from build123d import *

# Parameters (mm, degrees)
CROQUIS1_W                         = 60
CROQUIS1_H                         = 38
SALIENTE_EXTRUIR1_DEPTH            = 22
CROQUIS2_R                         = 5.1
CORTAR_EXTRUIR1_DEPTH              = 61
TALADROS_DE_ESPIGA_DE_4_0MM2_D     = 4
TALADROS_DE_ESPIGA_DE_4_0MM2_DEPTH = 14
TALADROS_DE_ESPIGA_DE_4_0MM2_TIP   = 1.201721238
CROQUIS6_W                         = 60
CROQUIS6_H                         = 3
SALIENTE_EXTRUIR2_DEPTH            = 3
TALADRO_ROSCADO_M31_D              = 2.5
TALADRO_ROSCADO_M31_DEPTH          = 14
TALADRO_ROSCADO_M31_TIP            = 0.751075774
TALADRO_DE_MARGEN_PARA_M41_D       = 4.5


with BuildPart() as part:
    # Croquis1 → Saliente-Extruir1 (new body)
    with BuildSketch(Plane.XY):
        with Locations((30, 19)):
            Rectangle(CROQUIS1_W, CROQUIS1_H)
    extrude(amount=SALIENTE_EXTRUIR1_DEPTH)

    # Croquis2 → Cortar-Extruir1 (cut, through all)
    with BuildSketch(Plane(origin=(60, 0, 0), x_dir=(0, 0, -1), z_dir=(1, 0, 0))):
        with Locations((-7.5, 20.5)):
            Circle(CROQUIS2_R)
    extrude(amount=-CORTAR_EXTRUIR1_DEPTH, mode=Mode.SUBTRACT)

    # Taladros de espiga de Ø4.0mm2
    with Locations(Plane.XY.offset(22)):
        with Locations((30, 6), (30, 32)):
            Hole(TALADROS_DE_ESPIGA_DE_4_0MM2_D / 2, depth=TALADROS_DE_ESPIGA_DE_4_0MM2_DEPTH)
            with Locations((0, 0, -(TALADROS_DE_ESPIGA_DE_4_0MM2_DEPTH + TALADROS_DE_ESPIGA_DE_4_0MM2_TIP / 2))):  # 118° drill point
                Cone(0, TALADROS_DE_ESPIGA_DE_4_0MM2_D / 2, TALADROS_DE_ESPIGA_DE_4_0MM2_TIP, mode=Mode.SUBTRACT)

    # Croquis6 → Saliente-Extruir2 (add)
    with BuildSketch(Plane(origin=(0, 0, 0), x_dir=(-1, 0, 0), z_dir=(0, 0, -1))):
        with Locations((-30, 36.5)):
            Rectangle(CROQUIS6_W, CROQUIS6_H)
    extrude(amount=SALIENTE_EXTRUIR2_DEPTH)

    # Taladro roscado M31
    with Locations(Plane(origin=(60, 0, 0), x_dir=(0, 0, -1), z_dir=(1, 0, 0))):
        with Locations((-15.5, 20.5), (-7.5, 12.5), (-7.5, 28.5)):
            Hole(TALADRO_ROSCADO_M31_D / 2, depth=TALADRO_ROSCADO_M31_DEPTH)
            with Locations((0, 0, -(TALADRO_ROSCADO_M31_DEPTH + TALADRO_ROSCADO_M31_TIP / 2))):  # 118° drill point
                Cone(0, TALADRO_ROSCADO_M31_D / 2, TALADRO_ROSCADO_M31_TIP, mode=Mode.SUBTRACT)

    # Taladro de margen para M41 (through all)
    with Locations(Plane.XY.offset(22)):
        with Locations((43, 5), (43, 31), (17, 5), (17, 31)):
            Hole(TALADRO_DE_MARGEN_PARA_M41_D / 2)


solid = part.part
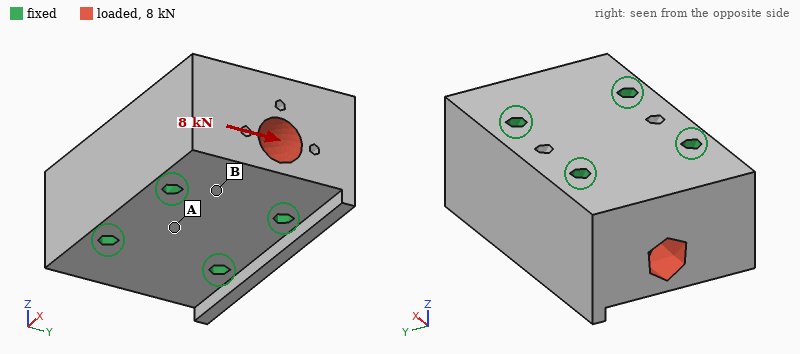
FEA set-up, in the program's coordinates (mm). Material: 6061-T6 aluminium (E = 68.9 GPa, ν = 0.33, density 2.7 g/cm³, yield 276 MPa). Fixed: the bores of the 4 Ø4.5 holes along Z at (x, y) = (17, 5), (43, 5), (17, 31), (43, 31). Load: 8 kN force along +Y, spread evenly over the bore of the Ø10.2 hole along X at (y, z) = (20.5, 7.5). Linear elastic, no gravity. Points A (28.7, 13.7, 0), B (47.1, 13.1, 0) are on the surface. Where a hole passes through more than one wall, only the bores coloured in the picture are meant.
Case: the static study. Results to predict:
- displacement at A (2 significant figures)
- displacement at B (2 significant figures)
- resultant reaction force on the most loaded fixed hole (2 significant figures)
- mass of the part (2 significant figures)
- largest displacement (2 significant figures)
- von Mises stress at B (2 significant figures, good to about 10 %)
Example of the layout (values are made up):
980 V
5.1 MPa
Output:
1.2 µm
1.1 µm
2.2 kN
120 g
2.9 µm
6.6 MPa
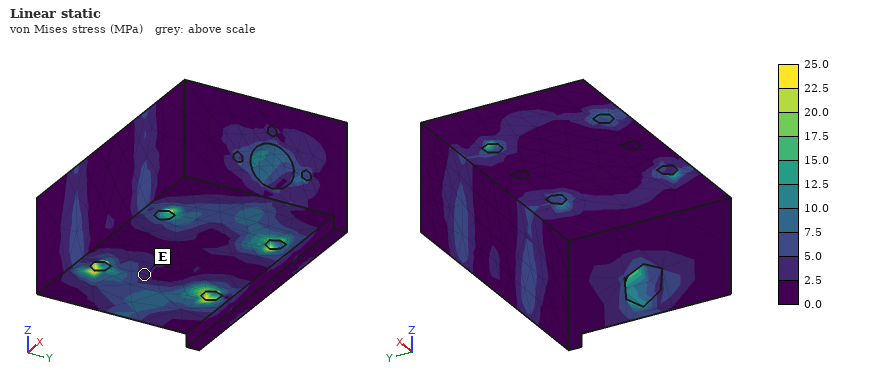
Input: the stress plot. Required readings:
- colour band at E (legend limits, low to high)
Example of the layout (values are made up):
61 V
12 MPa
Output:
2.5 to 5.0 MPa
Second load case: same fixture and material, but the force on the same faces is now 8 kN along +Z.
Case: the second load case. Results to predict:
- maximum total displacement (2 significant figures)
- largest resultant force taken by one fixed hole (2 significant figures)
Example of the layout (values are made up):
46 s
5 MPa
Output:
5.4 µm
2.3 kN
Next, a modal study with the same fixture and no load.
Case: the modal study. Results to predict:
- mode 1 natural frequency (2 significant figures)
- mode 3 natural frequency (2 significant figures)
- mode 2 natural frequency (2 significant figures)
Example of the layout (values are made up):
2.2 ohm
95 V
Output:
31 kHz
35 kHz
32 kHz
